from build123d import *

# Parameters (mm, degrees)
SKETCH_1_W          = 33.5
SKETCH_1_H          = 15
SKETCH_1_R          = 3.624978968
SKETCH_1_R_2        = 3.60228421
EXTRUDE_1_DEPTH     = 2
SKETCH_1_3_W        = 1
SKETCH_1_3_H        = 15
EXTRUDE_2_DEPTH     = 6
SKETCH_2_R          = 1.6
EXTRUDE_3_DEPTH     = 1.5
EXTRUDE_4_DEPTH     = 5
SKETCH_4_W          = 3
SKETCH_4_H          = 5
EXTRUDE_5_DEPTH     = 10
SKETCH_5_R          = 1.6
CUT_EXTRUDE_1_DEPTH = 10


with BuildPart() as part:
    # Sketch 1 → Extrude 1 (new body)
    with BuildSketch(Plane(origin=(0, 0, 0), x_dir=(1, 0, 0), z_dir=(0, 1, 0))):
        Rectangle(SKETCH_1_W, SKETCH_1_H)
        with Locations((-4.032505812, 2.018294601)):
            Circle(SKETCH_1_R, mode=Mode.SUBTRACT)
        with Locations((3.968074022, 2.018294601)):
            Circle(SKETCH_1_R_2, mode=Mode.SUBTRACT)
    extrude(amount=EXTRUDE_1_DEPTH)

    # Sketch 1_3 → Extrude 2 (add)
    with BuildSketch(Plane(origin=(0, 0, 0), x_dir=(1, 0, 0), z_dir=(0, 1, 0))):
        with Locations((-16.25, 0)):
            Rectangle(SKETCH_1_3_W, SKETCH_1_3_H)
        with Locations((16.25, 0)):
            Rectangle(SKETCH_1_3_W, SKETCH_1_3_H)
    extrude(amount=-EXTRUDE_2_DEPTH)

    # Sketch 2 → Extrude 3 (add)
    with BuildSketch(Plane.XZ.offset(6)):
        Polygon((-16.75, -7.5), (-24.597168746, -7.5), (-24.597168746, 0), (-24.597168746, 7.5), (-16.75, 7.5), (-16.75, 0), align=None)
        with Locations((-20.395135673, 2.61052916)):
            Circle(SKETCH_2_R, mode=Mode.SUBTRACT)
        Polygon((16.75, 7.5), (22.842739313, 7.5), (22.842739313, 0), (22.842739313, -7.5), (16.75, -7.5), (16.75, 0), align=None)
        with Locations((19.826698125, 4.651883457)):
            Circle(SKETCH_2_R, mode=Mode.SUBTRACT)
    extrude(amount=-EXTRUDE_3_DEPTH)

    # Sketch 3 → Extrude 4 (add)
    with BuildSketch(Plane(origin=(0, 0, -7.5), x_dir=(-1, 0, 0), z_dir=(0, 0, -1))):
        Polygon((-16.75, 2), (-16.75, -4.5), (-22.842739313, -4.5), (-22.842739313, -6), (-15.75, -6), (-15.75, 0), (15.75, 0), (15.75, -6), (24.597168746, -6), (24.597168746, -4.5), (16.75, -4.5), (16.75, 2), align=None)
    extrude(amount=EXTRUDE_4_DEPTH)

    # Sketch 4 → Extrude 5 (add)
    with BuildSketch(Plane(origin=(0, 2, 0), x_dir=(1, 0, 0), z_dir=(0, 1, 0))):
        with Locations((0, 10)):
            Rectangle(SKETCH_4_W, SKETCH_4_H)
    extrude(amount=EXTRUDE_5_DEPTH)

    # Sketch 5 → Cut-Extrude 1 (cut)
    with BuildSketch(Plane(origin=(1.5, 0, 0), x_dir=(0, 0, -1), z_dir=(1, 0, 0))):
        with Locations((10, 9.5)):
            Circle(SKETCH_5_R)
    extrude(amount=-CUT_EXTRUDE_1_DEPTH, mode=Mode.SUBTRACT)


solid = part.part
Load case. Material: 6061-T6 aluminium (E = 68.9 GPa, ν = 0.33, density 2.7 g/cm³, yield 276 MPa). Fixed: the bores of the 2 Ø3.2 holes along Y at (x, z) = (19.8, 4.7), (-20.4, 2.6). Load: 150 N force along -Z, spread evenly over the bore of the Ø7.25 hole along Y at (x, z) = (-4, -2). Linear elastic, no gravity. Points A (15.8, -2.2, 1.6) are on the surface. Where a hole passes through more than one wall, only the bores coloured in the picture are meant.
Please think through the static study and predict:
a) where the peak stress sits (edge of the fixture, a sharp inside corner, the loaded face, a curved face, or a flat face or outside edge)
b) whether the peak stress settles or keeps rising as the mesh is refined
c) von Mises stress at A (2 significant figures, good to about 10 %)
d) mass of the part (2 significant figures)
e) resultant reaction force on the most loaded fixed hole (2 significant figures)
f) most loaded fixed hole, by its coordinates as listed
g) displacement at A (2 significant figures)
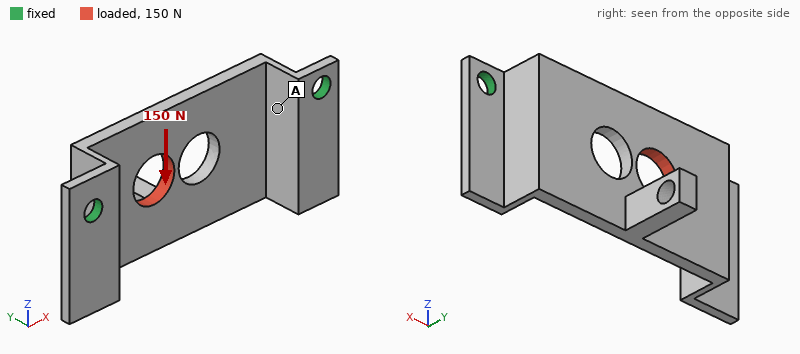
edge of the fixture
keeps rising
16 MPa
5.2 g
94 N
(-20.4, 2.6)
13 µm
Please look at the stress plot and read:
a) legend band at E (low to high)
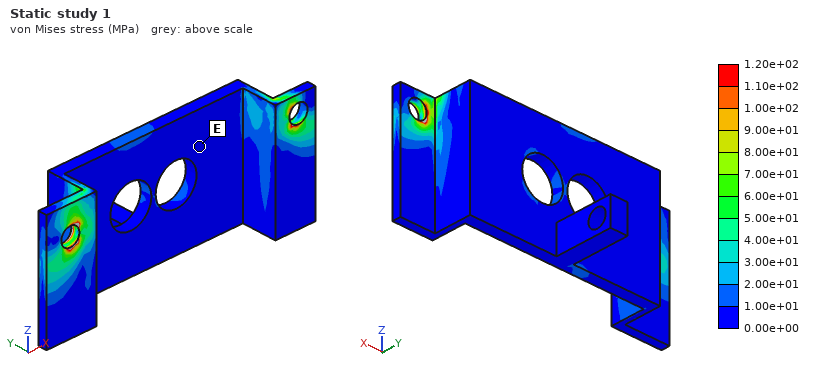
0.00e+00 to 1.00e+01 MPa
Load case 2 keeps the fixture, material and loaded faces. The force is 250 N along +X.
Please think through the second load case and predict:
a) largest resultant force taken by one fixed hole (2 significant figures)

130 N
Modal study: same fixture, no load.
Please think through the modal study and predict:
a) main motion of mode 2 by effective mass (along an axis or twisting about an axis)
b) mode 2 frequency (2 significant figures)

along X
6100 Hz
